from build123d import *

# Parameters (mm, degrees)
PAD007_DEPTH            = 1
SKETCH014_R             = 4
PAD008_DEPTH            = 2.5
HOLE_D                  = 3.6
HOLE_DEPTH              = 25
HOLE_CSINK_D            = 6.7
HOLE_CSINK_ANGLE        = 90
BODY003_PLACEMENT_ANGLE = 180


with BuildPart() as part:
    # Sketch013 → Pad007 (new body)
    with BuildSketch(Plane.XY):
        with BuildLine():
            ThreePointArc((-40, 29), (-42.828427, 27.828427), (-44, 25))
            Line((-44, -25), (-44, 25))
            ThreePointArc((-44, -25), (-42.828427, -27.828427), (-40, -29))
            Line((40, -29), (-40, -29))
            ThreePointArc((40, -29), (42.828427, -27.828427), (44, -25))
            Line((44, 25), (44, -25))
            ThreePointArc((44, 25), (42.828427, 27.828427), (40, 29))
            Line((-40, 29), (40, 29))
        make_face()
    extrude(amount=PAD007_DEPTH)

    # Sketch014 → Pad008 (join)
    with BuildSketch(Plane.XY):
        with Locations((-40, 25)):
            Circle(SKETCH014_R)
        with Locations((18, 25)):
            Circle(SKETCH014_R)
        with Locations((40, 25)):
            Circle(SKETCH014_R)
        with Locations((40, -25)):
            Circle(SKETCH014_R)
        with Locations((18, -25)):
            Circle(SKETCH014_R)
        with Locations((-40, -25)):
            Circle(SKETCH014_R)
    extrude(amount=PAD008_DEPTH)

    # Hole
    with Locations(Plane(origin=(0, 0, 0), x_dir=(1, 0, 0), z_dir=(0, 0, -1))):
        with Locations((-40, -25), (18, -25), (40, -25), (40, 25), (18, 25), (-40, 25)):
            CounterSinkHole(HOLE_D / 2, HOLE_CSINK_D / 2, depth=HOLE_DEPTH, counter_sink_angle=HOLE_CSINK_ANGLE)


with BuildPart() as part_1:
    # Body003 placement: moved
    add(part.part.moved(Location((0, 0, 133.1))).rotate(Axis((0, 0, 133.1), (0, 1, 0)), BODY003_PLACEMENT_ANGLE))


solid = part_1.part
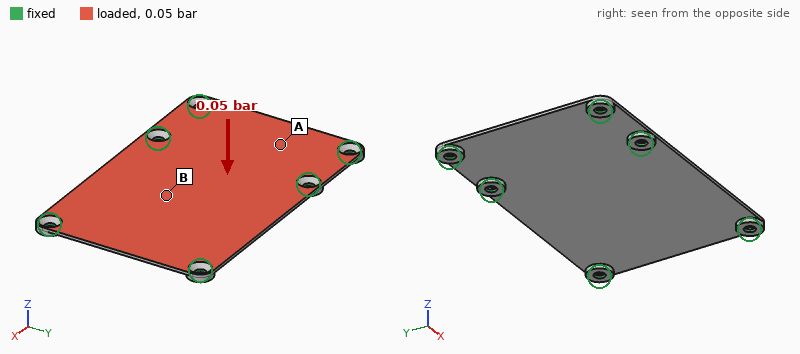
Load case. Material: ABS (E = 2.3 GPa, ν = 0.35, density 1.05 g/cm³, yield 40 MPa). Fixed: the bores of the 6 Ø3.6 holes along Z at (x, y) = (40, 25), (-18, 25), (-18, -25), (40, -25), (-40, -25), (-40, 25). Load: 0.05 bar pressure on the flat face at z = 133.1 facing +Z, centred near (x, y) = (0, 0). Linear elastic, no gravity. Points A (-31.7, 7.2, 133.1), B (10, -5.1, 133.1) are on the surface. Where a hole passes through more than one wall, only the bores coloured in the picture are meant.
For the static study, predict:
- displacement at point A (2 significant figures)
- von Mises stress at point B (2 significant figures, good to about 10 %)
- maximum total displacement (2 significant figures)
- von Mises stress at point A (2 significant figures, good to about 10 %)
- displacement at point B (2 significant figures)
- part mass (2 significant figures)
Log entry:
0.24 mm
4.2 MPa
1.1 mm
1.8 MPa
1.1 mm
5.5 g
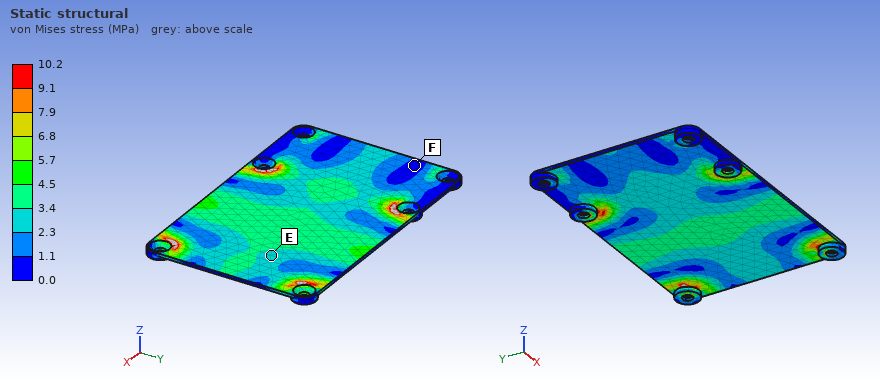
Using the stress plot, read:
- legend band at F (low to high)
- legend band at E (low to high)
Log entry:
0.0 to 1.1 MPa
2.3 to 3.4 MPa
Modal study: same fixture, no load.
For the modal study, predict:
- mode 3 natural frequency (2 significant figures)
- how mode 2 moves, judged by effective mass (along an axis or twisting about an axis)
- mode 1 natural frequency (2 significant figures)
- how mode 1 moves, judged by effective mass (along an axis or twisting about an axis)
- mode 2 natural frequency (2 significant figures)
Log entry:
750 Hz
twisting about X
410 Hz
along Z
620 Hz
